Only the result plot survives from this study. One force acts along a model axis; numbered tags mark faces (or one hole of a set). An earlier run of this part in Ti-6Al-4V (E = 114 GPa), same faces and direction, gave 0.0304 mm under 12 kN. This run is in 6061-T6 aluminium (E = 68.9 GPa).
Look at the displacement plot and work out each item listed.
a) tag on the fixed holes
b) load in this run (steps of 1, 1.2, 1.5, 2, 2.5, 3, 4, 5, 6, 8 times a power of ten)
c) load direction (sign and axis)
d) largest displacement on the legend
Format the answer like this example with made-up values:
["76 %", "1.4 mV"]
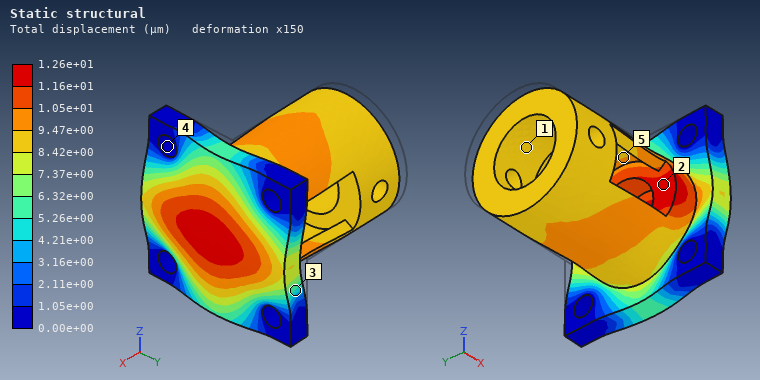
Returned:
["4", "3 kN", "+X", "1.26e+01 µm"]
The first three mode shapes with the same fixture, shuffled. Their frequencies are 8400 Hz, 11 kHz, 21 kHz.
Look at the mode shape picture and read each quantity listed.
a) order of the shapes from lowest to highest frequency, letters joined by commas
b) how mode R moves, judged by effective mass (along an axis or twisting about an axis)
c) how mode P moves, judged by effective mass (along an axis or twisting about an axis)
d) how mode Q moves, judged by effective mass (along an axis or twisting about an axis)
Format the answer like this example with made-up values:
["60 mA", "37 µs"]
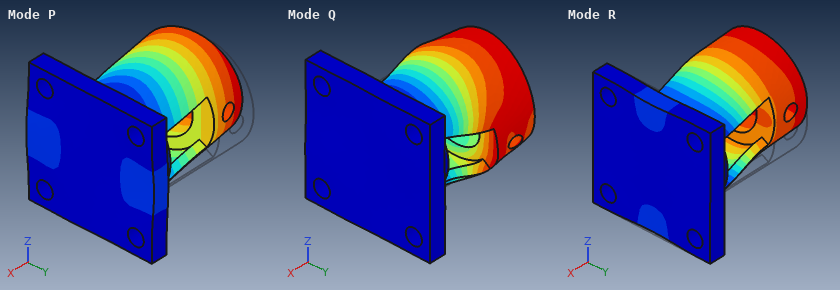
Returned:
["R, P, Q", "along Z", "along Y", "twisting about X"]
